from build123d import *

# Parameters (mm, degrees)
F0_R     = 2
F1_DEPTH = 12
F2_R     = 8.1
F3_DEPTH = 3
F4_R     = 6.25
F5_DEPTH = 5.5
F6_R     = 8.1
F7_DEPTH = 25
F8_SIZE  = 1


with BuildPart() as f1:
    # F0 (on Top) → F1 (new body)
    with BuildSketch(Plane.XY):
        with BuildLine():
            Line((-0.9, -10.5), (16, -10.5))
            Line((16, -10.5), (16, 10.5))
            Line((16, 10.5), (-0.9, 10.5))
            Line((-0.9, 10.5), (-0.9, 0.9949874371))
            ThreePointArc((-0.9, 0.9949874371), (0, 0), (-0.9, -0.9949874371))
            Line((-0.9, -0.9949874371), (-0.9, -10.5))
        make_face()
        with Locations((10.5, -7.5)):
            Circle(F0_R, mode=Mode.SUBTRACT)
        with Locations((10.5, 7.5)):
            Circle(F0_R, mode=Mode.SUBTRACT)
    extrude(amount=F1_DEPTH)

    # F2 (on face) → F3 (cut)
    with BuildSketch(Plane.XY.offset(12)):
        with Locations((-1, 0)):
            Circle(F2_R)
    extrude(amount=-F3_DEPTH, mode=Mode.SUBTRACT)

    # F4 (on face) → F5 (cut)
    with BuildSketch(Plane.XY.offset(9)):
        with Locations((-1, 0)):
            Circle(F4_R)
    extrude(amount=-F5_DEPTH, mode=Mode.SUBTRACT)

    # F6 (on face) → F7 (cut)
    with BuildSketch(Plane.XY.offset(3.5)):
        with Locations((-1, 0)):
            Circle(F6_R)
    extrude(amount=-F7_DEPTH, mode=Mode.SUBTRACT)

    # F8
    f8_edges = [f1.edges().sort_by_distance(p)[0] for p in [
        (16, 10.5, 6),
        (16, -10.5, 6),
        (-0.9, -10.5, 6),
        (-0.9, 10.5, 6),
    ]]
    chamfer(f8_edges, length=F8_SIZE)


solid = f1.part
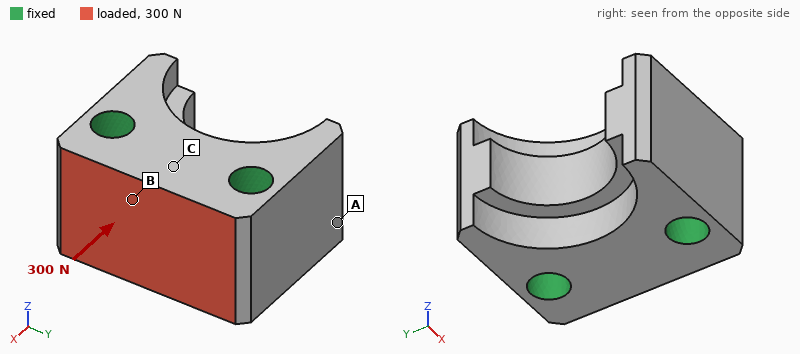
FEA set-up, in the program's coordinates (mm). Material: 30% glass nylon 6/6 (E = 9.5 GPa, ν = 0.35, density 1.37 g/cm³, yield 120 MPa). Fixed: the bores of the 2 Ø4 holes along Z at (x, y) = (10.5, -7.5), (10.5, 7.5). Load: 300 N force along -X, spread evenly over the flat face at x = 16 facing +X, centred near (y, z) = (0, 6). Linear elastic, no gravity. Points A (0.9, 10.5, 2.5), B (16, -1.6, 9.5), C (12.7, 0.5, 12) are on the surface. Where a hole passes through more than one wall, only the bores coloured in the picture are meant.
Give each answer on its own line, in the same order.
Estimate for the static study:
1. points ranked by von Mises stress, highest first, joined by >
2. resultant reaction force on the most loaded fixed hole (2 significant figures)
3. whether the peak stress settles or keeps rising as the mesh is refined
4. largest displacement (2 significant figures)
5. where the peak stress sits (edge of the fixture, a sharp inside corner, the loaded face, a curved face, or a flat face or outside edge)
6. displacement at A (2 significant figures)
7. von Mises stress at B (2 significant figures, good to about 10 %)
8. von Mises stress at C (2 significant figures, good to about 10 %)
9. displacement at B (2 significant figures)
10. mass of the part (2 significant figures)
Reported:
B > C > A
150 N
keeps rising
1.7 µm
edge of the fixture
0.71 µm
1.3 MPa
0.80 MPa
1.4 µm
4.0 g
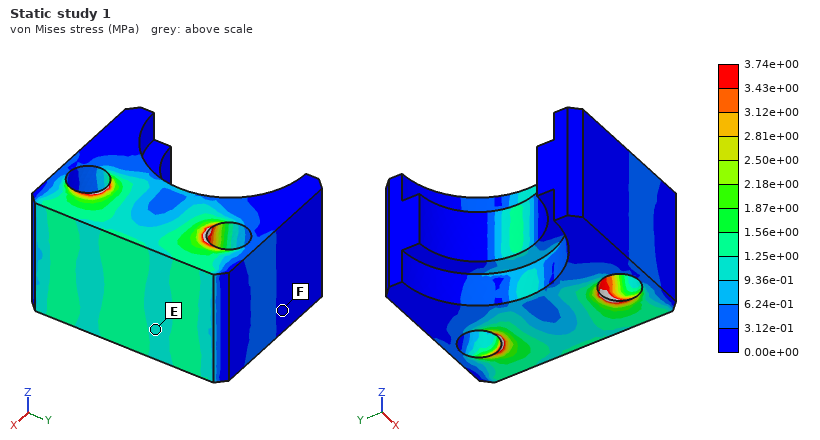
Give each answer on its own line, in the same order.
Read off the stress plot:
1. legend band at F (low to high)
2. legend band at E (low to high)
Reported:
0.00e+00 to 3.12e-01 MPa
9.36e-01 to 1.25e+00 MPa
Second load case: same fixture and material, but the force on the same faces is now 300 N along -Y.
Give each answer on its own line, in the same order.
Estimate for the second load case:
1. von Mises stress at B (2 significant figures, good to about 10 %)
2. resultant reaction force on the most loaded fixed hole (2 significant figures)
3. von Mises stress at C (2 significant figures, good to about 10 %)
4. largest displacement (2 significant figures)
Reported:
2.3 MPa
170 N
1.8 MPa
2.2 µm
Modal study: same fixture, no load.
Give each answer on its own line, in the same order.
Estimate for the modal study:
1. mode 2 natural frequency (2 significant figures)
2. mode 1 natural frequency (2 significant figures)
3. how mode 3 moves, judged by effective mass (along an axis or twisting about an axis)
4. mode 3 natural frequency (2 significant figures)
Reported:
31 kHz
31 kHz
along Z
36 kHz
